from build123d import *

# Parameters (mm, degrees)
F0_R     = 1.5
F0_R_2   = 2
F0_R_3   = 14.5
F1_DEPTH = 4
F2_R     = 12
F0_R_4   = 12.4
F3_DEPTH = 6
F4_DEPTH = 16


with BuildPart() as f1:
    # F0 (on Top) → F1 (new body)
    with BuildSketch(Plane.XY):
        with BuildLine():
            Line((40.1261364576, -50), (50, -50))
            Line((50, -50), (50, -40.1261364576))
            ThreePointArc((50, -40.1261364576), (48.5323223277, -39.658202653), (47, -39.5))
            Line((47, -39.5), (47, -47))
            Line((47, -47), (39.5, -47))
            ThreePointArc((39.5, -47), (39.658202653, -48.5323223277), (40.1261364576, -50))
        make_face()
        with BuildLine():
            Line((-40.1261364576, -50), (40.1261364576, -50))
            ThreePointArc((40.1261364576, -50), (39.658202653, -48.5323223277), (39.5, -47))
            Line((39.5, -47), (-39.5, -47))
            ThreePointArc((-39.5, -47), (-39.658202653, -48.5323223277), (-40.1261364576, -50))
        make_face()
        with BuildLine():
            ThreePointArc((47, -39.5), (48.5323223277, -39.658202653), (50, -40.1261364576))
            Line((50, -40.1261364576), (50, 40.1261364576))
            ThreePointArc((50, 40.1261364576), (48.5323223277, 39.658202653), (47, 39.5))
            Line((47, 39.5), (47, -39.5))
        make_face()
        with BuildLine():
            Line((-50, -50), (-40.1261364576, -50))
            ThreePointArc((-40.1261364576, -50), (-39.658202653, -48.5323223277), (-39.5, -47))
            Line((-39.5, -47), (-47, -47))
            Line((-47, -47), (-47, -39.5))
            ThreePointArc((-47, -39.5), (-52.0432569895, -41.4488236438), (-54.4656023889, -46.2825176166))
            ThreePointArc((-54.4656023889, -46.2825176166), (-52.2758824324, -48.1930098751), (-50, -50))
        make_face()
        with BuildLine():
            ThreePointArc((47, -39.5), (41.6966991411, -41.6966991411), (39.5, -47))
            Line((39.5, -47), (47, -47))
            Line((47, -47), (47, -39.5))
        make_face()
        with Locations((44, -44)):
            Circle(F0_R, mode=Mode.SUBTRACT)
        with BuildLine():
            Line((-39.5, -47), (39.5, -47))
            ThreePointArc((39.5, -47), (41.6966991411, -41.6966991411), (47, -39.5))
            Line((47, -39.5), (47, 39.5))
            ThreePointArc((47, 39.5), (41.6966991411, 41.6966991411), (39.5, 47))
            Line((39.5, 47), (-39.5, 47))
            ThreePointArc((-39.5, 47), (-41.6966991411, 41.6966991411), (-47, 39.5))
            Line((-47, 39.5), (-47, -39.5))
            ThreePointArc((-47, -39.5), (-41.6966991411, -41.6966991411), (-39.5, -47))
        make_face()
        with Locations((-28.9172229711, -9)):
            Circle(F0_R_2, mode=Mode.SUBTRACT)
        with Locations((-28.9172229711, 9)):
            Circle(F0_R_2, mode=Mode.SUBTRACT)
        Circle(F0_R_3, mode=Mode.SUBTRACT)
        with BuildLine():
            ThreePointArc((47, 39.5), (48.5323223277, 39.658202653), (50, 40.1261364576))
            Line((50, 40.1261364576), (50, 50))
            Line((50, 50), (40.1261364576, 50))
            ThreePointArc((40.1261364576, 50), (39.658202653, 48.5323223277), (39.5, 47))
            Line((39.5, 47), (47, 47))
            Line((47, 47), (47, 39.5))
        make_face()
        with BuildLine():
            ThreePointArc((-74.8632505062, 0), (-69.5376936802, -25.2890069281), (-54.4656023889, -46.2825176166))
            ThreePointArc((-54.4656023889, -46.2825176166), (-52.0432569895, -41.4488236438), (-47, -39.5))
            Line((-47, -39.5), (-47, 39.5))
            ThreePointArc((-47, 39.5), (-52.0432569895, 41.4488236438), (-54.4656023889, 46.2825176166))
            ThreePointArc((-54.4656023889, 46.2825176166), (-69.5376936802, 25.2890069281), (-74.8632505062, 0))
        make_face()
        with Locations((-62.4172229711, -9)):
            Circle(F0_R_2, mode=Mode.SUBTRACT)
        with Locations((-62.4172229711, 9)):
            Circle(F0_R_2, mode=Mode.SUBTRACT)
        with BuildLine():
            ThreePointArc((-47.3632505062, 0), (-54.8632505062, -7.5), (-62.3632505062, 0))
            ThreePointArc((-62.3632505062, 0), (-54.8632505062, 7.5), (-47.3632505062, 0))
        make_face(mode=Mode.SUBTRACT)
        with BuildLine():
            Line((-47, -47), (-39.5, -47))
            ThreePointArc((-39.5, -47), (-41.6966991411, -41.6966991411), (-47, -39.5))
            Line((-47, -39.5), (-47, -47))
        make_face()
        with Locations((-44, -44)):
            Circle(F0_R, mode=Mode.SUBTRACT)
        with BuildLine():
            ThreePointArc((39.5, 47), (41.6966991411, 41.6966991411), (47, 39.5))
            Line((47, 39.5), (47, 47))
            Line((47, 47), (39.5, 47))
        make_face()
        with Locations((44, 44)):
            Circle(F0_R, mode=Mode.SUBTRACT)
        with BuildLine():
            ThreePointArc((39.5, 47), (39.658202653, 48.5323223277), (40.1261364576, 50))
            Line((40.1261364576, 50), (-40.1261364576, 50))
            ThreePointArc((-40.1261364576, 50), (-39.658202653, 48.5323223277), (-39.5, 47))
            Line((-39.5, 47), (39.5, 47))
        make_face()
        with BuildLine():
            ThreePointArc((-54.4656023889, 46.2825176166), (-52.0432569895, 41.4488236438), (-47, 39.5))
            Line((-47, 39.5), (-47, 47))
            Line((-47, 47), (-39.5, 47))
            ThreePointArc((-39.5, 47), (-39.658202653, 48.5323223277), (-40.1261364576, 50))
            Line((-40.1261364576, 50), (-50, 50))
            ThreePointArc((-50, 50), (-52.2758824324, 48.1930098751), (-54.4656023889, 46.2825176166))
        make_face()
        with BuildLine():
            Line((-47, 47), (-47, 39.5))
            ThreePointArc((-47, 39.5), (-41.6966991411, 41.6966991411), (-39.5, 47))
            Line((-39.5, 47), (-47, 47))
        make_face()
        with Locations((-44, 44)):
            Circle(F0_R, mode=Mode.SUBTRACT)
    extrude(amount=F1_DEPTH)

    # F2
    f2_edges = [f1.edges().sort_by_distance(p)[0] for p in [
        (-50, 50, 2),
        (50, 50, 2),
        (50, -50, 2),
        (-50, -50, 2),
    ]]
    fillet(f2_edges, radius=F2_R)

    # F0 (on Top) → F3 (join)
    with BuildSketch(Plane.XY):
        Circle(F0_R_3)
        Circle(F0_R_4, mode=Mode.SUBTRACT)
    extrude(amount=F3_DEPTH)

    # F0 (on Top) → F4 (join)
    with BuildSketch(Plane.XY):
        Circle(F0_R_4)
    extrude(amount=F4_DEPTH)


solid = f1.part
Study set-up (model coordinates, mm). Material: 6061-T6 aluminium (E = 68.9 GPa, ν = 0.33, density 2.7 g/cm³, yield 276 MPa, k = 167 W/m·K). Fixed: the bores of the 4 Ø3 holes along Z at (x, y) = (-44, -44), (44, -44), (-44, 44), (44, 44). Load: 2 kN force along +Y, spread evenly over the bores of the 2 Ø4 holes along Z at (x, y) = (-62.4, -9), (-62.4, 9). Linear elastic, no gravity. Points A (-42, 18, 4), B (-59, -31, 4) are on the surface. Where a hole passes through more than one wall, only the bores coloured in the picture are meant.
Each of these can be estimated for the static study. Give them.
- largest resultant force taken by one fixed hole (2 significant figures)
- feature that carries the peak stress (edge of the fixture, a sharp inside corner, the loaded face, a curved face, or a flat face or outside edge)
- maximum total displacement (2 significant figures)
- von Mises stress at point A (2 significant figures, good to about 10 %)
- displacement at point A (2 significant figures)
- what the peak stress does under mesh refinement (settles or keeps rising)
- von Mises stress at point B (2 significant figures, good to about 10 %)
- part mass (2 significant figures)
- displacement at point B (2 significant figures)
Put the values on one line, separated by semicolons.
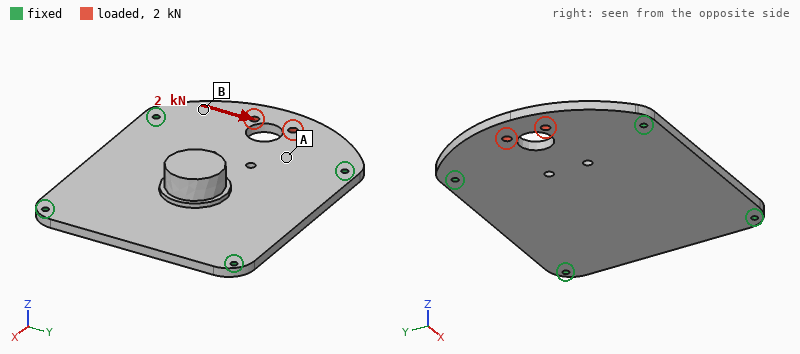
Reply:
1.0 kN; edge of the fixture; 14 µm; 3.8 MPa; 3.2 µm; keeps rising; 11 MPa; 140 g; 6.2 µm
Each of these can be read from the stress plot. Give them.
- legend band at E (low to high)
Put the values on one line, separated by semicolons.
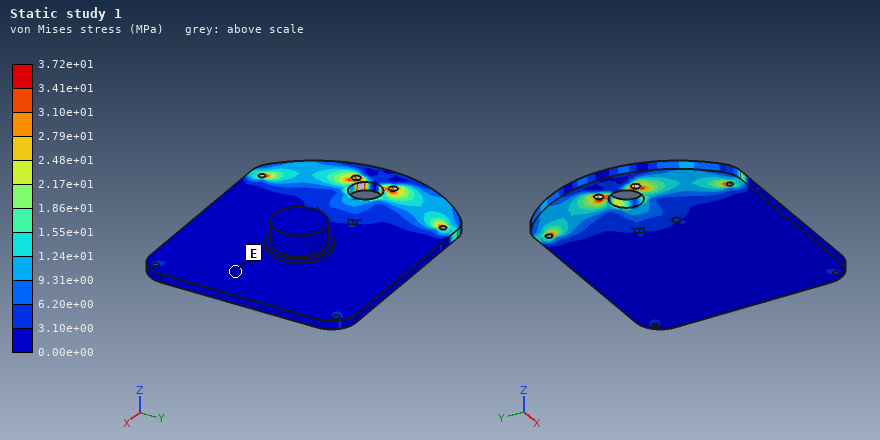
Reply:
0.00e+00 to 3.10e+00 MPa
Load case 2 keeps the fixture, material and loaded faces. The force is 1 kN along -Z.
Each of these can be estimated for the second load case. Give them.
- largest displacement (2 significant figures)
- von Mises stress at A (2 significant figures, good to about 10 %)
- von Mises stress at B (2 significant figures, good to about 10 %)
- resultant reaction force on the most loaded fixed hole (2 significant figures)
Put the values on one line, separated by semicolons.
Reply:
0.73 mm; 68 MPa; 57 MPa; 560 N
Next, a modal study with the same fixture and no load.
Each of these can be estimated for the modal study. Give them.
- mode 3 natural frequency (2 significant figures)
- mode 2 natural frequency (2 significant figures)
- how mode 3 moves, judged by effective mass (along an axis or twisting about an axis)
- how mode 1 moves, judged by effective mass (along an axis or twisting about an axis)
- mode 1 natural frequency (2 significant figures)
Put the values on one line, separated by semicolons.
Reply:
2700 Hz; 2000 Hz; twisting about X; along Z; 1500 Hz
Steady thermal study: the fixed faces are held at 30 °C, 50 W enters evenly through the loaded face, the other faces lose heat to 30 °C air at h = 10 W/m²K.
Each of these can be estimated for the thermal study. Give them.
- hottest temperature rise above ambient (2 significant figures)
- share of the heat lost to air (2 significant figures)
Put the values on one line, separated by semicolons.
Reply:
60 K; 6.8 %
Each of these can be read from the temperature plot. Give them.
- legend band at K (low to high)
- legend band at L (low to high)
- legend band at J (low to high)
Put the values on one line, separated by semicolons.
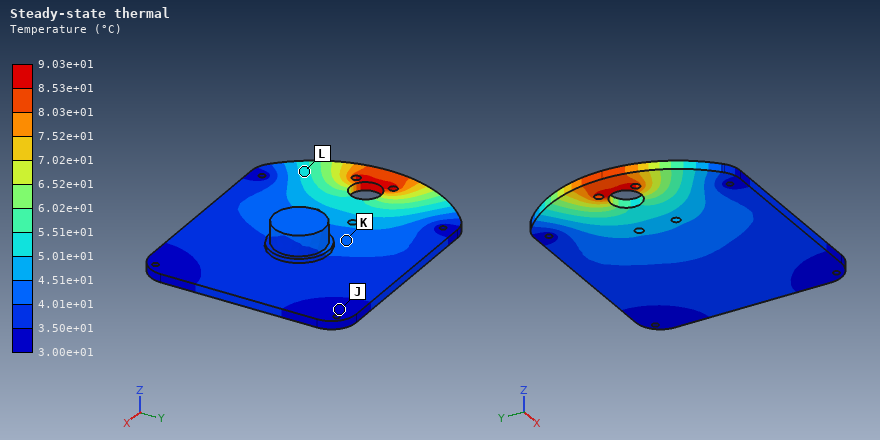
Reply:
4.01e+01 to 4.51e+01 °C; 5.01e+01 to 5.51e+01 °C; 3.00e+01 to 3.50e+01 °C
